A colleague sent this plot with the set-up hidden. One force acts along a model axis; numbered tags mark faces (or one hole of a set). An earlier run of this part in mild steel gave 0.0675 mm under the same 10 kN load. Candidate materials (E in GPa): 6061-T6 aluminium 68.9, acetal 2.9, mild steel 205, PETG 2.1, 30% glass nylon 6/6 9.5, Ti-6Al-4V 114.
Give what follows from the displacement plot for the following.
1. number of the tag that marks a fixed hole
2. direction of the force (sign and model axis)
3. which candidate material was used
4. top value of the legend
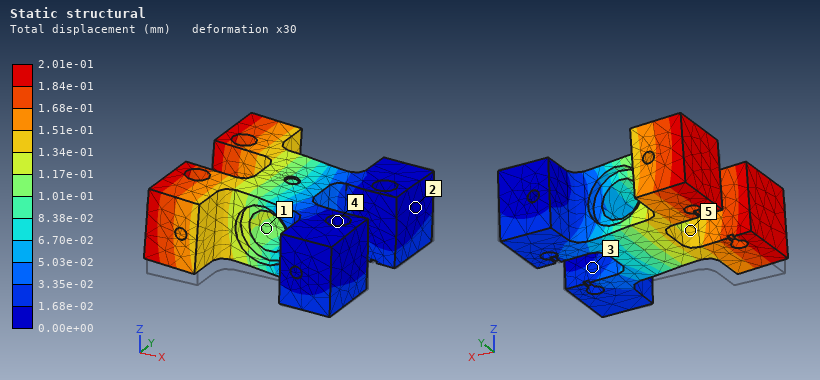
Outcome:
4
+Z
6061-T6 aluminium
2.01e-01 mm
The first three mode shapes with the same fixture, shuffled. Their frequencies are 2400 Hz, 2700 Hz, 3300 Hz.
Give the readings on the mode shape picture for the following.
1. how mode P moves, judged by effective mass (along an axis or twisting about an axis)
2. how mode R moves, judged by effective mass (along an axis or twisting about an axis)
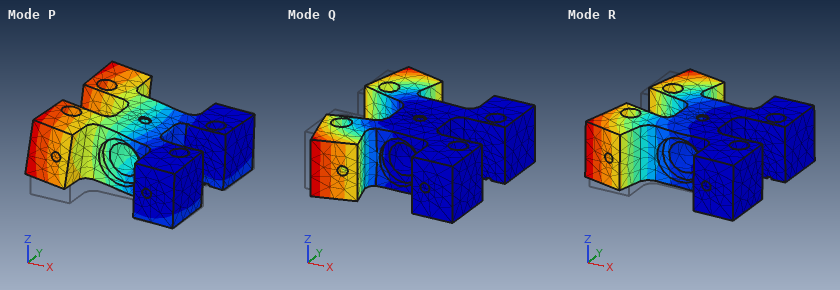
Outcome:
along Z
along Y
